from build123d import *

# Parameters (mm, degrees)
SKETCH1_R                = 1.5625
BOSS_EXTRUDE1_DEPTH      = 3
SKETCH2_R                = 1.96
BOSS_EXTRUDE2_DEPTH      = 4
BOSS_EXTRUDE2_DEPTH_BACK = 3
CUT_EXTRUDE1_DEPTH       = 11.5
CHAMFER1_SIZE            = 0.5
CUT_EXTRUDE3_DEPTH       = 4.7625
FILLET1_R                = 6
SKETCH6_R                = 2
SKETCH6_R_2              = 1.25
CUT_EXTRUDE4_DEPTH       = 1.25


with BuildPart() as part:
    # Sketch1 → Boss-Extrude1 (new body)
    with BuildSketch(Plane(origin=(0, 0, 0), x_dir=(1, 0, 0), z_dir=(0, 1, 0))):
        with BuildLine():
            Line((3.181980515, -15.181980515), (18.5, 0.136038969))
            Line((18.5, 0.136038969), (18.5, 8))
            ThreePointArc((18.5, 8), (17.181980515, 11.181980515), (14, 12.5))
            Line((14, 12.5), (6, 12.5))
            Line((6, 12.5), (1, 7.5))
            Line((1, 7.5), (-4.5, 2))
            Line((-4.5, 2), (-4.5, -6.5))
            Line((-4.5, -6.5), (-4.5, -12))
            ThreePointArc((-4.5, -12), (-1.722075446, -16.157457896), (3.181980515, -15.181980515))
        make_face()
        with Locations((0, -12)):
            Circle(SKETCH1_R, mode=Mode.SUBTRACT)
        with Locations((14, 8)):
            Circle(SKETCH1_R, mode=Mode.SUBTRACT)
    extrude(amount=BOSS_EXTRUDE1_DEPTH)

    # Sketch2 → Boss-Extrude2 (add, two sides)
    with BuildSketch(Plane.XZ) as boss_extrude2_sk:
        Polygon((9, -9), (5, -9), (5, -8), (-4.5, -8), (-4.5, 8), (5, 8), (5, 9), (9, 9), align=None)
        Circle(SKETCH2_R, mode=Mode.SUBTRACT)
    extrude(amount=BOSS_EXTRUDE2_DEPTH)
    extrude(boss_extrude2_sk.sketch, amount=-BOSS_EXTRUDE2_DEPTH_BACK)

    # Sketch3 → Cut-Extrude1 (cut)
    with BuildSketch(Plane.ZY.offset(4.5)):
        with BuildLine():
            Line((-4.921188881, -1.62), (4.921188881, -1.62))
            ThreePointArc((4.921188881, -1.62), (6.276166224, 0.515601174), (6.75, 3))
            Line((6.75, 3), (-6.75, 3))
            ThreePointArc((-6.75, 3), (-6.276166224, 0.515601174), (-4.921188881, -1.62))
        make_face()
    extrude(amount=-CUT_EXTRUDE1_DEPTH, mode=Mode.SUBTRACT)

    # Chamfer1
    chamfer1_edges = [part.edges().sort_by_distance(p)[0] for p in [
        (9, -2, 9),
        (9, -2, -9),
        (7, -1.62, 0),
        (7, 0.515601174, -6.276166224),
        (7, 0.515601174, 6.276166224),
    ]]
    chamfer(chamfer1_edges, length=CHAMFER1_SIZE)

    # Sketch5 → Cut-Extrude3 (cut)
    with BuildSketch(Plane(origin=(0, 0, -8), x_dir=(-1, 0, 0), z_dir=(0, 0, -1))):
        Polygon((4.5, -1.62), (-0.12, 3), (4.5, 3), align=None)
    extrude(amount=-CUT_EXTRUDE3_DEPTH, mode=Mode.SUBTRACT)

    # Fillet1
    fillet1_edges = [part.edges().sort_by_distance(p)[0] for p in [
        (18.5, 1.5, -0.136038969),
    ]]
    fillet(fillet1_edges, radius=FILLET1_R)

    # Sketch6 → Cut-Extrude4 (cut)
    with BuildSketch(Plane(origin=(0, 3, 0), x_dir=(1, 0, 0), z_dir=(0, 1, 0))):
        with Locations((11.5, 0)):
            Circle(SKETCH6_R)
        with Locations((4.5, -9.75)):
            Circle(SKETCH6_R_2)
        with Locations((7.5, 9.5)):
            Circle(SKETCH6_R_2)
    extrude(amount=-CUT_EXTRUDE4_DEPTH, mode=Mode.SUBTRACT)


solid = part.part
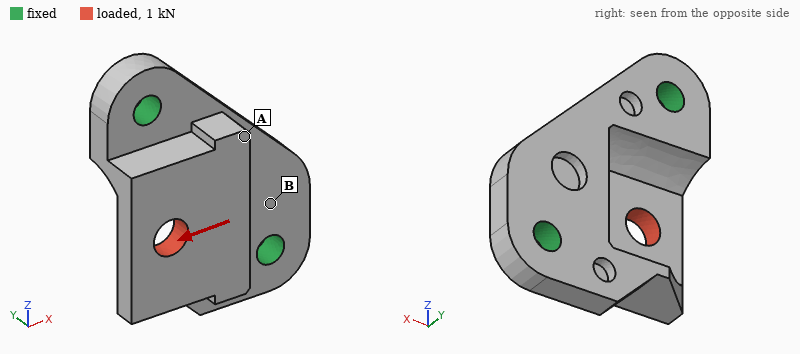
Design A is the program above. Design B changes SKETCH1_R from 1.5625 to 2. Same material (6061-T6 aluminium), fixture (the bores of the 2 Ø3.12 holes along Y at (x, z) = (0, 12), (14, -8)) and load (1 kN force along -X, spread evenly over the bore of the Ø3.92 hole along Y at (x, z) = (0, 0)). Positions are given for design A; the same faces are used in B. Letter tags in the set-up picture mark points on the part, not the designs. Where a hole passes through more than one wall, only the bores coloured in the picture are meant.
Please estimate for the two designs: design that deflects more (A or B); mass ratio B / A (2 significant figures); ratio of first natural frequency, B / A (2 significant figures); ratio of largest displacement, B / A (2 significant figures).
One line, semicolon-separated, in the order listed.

A; 0.98; 1.1; 0.86
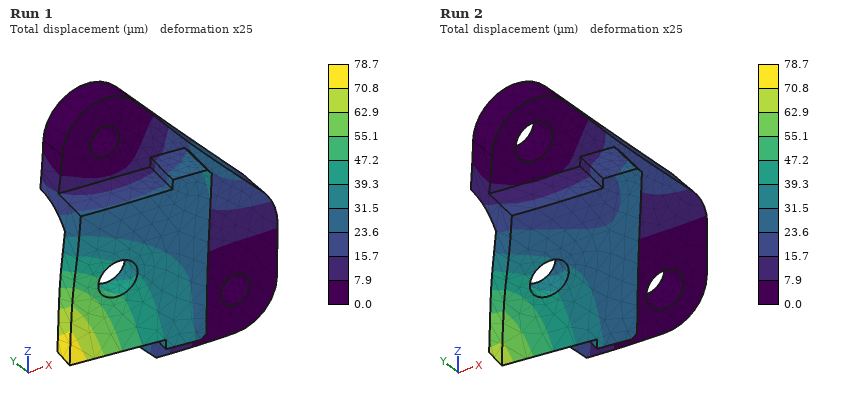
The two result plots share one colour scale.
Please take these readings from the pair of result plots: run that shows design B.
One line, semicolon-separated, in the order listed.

Run 2
